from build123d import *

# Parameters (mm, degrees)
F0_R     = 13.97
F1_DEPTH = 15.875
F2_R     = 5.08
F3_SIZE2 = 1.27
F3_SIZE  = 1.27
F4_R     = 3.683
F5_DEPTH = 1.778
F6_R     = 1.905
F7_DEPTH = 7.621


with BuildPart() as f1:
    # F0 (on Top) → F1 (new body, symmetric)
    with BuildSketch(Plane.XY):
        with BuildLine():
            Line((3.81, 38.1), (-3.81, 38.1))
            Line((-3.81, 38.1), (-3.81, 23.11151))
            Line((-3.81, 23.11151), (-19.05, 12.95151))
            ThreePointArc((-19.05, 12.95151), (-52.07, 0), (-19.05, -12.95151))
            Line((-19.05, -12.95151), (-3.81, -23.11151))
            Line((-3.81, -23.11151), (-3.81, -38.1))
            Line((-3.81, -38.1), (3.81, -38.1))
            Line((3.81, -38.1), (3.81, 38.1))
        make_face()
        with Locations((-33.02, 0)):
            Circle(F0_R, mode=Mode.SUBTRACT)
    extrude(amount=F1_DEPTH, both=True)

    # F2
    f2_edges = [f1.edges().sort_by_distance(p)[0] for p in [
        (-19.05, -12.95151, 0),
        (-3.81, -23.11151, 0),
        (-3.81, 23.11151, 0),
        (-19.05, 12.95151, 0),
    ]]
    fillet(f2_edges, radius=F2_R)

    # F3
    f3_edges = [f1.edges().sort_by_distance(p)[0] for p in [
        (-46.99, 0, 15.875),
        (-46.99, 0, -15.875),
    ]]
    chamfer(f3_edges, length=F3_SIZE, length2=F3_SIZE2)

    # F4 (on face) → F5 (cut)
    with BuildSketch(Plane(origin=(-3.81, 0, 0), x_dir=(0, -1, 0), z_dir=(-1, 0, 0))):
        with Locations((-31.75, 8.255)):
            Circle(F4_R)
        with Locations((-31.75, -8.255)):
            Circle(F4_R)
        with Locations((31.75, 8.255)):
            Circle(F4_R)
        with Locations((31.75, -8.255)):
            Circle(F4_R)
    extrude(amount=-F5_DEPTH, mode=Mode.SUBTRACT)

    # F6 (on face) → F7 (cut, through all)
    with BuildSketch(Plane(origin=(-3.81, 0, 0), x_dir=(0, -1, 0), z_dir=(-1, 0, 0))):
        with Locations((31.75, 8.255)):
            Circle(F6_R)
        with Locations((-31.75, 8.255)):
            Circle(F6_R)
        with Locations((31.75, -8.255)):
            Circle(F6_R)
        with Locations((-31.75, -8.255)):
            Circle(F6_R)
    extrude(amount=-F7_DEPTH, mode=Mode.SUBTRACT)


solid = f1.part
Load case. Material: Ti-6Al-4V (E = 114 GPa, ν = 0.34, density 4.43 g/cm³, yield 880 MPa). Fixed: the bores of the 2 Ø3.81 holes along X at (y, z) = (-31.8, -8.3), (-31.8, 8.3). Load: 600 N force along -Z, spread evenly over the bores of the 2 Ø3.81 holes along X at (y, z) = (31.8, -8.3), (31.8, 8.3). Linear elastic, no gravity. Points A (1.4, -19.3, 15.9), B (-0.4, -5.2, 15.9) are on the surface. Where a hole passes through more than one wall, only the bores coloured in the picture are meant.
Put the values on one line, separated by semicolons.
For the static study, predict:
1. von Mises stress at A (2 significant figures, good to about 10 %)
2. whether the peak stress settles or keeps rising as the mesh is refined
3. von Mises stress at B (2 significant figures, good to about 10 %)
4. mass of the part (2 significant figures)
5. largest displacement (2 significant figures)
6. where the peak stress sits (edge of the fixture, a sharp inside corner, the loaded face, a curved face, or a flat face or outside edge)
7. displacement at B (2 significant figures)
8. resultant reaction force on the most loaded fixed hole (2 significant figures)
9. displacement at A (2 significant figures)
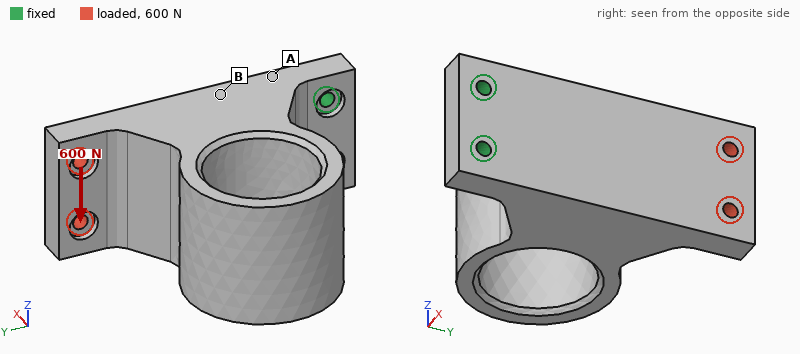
21 MPa; keeps rising; 9.4 MPa; 220 g; 34 µm; edge of the fixture; 12 µm; 2.0 kN; 6.6 µm
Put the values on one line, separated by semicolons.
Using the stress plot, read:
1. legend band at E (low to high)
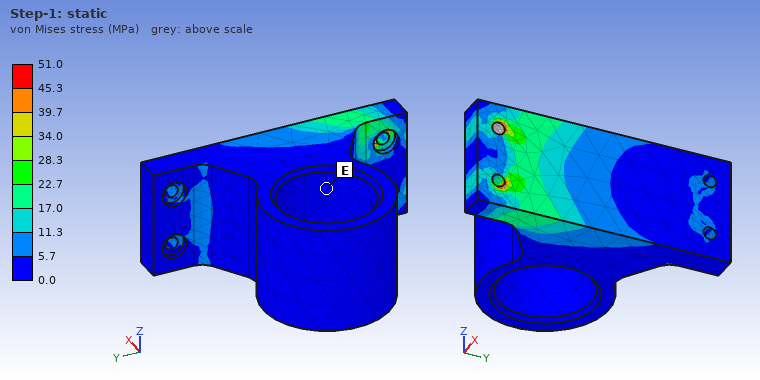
0.0 to 5.7 MPa
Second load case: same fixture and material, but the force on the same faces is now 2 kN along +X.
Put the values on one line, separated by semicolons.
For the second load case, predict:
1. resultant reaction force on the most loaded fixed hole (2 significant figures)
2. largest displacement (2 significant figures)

1.0 kN; 0.95 mm
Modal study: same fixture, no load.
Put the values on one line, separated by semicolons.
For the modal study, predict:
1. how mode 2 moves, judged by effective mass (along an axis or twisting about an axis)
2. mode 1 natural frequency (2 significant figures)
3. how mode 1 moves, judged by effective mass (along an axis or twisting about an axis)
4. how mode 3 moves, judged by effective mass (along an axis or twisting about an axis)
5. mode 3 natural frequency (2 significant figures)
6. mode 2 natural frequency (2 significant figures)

along Z; 820 Hz; along X; along Z; 3400 Hz; 2300 Hz
